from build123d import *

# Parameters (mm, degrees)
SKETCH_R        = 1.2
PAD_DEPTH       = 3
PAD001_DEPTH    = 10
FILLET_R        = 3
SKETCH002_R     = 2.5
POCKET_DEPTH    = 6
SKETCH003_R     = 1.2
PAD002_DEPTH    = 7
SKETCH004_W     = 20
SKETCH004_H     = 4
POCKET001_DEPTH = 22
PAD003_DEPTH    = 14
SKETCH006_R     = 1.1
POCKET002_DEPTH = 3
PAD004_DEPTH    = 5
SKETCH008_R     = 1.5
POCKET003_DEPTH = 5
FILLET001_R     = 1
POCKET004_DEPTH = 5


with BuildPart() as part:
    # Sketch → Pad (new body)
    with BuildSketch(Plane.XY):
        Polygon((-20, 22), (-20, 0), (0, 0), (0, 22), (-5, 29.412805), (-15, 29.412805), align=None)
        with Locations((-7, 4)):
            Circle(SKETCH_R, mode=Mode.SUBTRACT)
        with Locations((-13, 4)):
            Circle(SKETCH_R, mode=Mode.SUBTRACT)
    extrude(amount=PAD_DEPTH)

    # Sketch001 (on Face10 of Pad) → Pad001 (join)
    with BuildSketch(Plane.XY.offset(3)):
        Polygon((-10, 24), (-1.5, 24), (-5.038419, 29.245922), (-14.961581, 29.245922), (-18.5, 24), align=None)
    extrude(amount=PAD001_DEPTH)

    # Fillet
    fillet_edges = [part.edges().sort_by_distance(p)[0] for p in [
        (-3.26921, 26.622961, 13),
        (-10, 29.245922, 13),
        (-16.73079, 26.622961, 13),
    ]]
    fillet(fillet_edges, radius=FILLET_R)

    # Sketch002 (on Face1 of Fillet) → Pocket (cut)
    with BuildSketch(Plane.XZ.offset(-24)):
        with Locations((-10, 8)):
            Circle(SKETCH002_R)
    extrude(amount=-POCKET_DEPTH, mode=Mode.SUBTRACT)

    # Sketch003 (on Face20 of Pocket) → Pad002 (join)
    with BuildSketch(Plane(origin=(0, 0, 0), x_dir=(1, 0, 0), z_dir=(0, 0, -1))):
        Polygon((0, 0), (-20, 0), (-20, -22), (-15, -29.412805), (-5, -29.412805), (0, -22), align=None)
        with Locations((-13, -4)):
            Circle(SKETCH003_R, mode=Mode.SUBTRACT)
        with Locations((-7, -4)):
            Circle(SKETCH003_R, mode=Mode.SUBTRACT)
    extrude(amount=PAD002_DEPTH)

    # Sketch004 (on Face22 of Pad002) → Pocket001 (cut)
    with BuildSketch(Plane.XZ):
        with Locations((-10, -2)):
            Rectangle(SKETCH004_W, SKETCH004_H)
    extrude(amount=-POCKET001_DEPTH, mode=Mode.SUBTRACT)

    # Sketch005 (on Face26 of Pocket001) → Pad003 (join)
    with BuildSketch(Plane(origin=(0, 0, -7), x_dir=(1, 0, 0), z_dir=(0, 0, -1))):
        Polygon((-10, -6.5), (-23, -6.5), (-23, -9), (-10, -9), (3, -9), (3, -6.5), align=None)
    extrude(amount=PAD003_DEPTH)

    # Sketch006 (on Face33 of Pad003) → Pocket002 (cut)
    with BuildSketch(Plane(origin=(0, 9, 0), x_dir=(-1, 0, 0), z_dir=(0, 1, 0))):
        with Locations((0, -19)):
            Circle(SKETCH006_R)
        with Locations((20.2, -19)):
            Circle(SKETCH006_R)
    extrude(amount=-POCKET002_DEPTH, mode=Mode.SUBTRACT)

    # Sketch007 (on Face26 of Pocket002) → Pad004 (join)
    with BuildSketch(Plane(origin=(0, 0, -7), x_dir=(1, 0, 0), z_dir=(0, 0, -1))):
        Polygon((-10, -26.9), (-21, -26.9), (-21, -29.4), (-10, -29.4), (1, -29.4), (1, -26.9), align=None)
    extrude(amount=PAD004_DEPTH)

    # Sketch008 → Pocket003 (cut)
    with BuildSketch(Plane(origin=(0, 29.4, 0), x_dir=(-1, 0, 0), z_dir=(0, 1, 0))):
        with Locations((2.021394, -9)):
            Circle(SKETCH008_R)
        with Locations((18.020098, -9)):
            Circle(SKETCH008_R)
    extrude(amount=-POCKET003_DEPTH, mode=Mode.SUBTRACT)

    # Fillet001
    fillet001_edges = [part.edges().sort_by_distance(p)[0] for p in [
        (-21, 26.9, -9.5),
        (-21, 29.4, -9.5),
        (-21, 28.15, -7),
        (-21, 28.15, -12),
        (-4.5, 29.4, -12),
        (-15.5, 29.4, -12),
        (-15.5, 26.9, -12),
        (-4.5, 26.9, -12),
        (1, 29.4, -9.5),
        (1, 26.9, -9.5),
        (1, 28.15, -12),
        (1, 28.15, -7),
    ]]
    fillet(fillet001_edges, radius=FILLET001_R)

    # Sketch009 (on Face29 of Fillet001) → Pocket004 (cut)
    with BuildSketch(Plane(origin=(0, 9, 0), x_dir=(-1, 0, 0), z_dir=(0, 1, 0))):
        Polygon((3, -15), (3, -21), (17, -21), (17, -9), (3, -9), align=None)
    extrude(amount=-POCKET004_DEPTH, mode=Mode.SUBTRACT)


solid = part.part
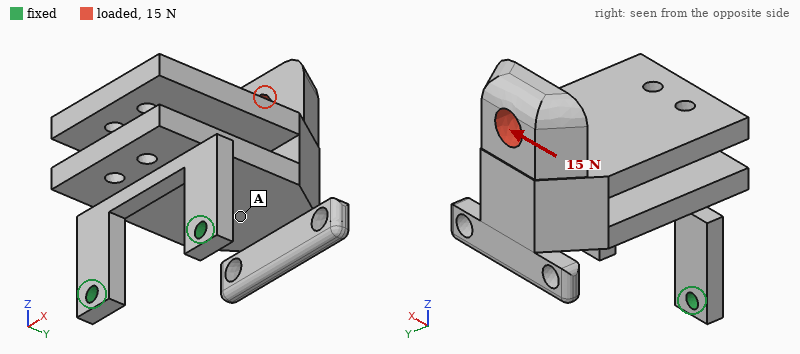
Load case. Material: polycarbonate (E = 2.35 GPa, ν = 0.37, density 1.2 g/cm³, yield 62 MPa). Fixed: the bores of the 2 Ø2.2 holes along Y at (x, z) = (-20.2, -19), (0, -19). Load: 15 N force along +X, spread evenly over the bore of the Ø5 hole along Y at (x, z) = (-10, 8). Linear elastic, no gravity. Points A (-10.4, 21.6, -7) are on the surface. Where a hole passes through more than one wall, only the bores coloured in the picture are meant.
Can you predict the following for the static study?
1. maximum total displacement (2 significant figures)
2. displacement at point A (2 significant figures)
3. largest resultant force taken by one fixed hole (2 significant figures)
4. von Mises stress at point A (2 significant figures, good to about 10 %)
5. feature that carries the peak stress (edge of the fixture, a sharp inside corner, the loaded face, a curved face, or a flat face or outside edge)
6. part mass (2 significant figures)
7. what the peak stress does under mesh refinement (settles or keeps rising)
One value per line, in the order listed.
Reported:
0.50 mm
0.21 mm
21 N
1.8 MPa
edge of the fixture
5.9 g
keeps rising
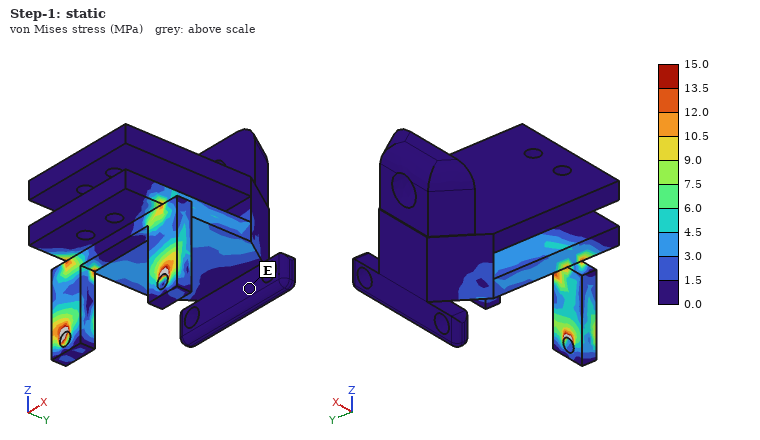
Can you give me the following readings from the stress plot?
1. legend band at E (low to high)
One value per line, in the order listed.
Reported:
0.0 to 1.5 MPa
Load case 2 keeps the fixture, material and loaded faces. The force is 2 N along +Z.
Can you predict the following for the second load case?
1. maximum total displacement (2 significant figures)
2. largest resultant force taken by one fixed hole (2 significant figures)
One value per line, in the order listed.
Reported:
0.51 mm
1.1 N
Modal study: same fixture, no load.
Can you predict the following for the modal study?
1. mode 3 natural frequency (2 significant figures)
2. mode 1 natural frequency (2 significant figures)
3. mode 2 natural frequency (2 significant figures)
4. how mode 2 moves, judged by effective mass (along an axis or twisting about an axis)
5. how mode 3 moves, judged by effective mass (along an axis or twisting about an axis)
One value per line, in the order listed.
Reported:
860 Hz
190 Hz
610 Hz
along X
along Z
